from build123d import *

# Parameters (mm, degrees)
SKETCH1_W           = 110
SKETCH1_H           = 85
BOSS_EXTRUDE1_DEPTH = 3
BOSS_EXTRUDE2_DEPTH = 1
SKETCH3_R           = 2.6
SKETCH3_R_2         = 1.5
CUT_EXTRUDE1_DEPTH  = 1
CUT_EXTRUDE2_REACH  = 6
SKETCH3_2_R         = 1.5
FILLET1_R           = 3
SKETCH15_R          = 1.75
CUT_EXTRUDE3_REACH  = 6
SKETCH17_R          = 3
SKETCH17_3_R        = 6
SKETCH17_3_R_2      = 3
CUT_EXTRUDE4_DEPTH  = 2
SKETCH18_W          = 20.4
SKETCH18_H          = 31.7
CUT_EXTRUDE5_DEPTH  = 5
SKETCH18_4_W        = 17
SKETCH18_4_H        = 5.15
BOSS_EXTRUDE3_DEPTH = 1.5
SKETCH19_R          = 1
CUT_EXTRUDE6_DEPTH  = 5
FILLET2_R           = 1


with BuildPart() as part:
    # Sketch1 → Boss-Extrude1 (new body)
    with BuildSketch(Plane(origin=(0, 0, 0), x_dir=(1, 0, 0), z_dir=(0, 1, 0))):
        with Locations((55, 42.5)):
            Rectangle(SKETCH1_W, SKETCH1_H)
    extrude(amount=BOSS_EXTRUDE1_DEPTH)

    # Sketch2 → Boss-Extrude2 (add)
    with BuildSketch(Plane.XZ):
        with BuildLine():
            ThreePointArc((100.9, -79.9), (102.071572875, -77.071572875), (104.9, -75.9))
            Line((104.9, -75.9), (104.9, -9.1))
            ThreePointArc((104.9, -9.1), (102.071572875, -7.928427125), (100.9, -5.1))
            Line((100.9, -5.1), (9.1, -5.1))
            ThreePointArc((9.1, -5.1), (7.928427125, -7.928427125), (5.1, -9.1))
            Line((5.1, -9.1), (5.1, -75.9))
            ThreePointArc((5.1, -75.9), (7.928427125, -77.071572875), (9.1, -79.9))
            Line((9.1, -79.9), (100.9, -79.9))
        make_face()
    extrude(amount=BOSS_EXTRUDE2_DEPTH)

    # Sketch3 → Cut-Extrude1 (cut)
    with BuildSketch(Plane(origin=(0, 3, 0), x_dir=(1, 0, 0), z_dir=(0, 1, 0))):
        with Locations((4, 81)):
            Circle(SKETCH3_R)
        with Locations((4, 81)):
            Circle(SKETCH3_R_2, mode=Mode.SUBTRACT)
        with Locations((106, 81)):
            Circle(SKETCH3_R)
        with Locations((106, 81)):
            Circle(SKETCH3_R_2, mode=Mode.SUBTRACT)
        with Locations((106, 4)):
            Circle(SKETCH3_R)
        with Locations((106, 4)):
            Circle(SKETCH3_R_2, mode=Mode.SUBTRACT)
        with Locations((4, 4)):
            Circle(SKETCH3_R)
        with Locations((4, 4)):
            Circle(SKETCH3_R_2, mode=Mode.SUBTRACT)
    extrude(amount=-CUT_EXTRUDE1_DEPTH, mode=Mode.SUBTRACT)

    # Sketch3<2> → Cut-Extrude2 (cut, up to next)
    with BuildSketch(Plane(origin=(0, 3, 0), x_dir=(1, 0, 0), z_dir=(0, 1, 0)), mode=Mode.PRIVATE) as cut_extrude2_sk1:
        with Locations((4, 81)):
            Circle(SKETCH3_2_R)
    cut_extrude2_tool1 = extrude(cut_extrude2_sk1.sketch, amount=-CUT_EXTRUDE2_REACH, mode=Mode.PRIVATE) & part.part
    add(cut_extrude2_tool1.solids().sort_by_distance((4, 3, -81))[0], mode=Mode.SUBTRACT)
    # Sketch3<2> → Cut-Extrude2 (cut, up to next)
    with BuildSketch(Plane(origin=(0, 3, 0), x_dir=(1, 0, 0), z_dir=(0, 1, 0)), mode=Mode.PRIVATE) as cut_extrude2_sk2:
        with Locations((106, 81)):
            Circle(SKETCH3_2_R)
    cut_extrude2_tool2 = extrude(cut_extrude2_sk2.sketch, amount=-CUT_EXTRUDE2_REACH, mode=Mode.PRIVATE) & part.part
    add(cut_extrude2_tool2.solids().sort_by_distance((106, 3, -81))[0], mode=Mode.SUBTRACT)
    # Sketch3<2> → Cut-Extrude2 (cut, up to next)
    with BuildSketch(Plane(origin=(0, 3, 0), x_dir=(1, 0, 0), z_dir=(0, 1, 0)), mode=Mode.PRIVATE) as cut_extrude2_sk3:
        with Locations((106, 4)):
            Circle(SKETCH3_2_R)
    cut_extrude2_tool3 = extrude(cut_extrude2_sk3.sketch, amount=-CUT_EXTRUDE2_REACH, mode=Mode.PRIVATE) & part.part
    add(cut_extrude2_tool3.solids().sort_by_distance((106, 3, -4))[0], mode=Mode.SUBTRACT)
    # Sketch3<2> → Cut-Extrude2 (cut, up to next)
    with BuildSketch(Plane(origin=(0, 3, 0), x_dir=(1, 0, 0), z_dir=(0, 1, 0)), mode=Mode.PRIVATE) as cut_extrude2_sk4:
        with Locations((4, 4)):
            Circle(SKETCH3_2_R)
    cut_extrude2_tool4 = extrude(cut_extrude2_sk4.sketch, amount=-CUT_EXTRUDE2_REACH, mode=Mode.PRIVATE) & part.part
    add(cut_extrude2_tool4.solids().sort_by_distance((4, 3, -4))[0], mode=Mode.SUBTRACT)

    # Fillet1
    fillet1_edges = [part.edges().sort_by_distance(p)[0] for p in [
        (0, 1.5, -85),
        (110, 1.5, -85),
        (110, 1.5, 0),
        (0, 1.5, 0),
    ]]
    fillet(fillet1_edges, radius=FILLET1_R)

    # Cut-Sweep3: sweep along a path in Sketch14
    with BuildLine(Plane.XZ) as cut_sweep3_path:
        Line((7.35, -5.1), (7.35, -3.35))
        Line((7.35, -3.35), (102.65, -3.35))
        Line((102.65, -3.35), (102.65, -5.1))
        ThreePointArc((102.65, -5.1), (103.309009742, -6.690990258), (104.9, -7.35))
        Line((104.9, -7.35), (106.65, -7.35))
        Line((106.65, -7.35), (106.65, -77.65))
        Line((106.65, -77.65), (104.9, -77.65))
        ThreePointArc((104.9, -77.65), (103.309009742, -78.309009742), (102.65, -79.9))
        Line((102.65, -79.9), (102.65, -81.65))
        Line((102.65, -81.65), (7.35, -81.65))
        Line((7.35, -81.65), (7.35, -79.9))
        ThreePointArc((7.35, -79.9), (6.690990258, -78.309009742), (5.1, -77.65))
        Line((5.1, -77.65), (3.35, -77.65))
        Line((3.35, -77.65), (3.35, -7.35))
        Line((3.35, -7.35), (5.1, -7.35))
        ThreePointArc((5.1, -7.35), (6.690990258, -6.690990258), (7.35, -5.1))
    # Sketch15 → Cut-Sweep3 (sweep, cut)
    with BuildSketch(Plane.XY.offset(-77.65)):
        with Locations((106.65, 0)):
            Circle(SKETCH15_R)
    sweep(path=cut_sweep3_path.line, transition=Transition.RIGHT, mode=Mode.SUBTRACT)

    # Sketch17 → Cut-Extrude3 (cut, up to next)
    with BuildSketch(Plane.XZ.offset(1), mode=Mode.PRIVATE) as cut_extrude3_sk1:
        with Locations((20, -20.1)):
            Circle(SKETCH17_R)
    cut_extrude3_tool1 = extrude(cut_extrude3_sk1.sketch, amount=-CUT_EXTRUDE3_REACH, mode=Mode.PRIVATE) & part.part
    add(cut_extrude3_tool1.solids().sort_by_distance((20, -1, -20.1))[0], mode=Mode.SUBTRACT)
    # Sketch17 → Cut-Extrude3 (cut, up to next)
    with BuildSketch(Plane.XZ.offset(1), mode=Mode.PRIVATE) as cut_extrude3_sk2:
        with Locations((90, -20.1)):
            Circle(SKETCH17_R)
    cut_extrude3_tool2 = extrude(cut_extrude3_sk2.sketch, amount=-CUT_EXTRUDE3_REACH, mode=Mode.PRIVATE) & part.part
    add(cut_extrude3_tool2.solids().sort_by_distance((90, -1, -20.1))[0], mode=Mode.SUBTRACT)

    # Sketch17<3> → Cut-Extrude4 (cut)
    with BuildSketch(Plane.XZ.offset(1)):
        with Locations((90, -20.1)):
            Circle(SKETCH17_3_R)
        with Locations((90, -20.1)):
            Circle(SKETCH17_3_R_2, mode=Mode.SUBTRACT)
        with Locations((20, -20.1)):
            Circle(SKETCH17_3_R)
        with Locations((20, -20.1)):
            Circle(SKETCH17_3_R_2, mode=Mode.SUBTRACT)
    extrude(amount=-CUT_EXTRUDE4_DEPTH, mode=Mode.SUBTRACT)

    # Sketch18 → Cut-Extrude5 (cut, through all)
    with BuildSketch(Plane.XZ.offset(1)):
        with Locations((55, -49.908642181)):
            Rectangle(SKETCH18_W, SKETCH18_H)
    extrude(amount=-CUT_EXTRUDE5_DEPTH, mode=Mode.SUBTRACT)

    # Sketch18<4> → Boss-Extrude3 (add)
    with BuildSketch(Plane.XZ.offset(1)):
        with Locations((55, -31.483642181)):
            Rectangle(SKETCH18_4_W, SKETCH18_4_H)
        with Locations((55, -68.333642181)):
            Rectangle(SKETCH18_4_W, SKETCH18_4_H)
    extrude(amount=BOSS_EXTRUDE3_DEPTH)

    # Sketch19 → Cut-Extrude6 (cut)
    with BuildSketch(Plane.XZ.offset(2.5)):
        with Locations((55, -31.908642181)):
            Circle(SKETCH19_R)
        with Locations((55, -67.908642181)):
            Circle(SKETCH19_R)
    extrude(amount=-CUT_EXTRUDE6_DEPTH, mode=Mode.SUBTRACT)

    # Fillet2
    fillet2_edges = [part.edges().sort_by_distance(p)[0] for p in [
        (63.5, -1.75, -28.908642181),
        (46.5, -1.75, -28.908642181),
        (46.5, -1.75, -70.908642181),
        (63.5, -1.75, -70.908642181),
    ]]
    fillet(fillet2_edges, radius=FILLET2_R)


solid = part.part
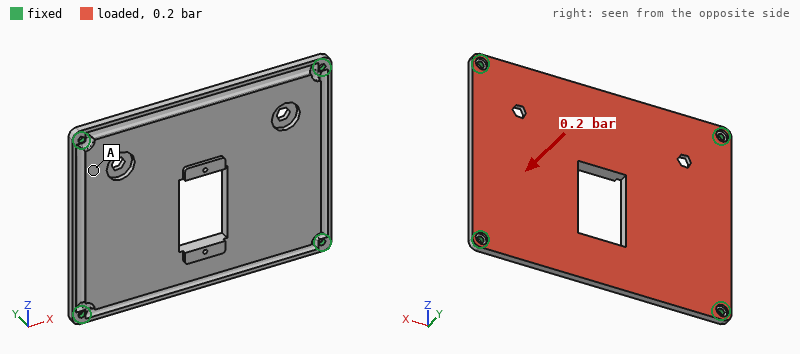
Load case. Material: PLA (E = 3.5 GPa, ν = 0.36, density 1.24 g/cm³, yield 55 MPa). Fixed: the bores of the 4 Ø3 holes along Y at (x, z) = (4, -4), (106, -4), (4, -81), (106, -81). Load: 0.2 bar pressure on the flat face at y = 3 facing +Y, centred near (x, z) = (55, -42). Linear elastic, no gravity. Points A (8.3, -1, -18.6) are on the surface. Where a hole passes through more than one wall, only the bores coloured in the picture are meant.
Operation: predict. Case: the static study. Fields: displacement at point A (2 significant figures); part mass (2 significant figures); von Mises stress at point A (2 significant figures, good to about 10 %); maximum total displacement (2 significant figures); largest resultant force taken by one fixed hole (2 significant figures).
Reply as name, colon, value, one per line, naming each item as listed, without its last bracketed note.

displacement at point A: 0.39 mm
part mass: 38 g
von Mises stress at point A: 6.0 MPa
maximum total displacement: 1.5 mm
largest resultant force taken by one fixed hole: 85 N
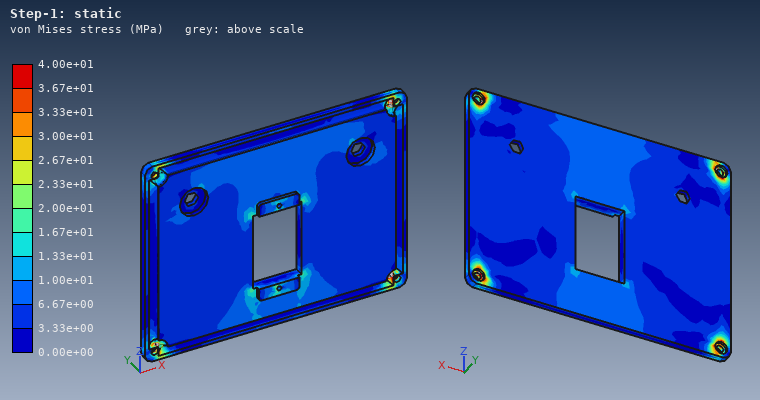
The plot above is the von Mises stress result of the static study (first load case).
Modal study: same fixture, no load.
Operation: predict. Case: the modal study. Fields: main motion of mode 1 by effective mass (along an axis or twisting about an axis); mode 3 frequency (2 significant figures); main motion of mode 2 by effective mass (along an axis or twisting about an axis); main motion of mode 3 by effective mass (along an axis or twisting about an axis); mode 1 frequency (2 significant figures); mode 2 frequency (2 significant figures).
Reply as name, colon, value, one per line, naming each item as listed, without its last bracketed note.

main motion of mode 1 by effective mass: along Y
mode 3 frequency: 750 Hz
main motion of mode 2 by effective mass: twisting about X
main motion of mode 3 by effective mass: twisting about Z
mode 1 frequency: 320 Hz
mode 2 frequency: 620 Hz
